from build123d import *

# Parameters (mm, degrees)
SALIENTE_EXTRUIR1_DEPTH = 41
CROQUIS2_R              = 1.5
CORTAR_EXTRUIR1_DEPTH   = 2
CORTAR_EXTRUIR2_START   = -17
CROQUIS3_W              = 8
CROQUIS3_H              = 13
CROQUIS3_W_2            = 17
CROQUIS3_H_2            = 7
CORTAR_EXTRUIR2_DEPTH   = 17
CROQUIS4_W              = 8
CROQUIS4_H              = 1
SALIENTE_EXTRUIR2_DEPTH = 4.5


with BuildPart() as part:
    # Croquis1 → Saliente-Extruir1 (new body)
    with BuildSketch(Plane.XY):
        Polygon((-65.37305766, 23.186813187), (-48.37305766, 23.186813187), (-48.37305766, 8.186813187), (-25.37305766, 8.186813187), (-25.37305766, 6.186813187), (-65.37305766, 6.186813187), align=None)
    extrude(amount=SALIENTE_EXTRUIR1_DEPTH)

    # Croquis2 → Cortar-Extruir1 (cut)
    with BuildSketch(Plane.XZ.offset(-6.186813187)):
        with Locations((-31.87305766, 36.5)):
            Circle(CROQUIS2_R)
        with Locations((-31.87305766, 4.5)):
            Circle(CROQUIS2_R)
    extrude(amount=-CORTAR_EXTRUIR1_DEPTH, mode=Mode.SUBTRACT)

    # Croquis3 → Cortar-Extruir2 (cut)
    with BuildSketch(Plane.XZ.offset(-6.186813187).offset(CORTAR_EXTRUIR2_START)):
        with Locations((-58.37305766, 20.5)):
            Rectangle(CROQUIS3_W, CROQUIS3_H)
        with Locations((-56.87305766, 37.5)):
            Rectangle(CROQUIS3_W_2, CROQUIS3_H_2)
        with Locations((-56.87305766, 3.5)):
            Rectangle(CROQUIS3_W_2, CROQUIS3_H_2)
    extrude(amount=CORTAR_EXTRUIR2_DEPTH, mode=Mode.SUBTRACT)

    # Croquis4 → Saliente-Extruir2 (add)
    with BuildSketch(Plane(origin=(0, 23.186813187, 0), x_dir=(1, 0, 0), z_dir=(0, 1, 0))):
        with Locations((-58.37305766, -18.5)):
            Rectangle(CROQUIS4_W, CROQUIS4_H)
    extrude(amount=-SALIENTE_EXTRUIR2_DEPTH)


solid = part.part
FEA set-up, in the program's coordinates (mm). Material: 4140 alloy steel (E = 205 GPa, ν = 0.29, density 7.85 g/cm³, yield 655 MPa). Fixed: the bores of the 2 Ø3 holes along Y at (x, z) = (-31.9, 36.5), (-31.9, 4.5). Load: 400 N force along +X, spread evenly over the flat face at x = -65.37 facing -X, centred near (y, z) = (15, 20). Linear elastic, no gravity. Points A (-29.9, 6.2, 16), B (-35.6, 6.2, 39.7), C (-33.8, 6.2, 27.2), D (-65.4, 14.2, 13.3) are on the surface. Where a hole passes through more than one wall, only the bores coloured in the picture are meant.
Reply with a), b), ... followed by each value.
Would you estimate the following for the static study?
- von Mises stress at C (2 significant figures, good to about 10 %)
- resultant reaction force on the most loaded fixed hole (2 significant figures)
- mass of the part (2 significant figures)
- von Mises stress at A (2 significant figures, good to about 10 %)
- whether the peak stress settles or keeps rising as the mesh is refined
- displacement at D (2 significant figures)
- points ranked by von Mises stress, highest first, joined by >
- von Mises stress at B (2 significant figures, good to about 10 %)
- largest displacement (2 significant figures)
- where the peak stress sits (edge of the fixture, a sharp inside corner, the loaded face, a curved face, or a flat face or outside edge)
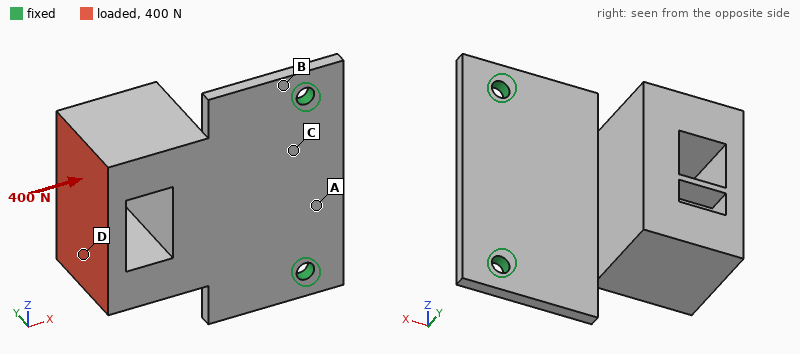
a) 62 MPa
b) 210 N
c) 62 g
d) 34 MPa
e) keeps rising
f) 0.28 mm
g) B > C > A > D
h) 130 MPa
i) 0.32 mm
j) edge of the fixture
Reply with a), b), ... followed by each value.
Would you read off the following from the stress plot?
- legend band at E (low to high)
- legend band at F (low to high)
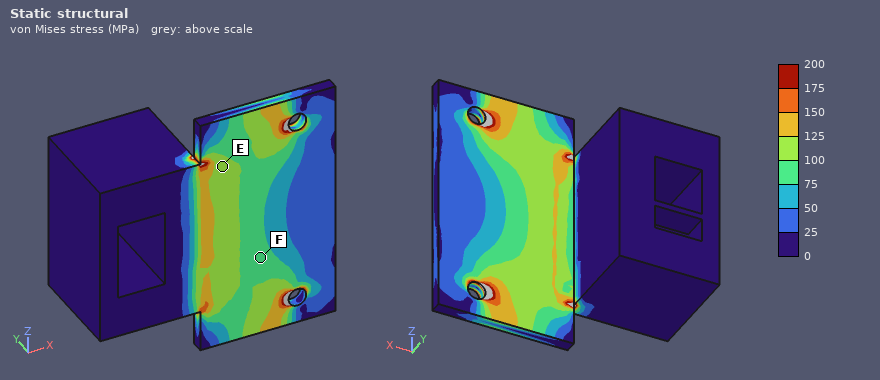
a) 100 to 125 MPa
b) 75 to 100 MPa
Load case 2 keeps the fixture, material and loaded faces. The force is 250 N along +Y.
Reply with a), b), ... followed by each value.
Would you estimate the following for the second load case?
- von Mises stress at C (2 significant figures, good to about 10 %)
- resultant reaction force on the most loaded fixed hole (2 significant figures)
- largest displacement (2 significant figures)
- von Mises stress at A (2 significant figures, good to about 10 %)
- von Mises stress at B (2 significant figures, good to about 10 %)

a) 160 MPa
b) 130 N
c) 0.69 mm
d) 86 MPa
e) 360 MPa
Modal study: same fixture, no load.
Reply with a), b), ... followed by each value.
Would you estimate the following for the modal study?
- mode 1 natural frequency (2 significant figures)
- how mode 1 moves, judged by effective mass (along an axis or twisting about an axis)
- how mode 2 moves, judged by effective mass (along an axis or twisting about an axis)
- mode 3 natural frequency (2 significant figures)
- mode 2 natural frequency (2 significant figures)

a) 610 Hz
b) along Y
c) along Z
d) 3500 Hz
e) 2200 Hz
